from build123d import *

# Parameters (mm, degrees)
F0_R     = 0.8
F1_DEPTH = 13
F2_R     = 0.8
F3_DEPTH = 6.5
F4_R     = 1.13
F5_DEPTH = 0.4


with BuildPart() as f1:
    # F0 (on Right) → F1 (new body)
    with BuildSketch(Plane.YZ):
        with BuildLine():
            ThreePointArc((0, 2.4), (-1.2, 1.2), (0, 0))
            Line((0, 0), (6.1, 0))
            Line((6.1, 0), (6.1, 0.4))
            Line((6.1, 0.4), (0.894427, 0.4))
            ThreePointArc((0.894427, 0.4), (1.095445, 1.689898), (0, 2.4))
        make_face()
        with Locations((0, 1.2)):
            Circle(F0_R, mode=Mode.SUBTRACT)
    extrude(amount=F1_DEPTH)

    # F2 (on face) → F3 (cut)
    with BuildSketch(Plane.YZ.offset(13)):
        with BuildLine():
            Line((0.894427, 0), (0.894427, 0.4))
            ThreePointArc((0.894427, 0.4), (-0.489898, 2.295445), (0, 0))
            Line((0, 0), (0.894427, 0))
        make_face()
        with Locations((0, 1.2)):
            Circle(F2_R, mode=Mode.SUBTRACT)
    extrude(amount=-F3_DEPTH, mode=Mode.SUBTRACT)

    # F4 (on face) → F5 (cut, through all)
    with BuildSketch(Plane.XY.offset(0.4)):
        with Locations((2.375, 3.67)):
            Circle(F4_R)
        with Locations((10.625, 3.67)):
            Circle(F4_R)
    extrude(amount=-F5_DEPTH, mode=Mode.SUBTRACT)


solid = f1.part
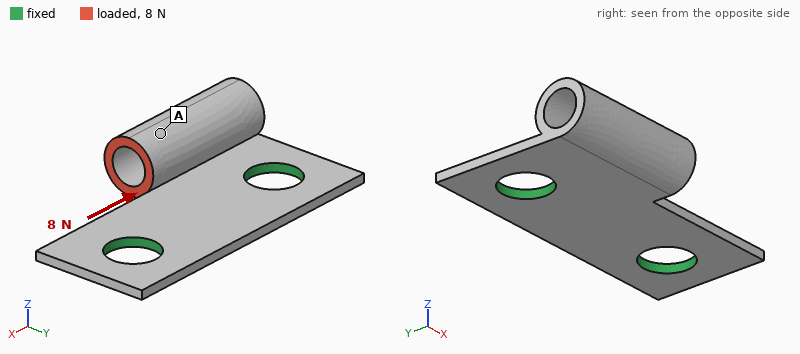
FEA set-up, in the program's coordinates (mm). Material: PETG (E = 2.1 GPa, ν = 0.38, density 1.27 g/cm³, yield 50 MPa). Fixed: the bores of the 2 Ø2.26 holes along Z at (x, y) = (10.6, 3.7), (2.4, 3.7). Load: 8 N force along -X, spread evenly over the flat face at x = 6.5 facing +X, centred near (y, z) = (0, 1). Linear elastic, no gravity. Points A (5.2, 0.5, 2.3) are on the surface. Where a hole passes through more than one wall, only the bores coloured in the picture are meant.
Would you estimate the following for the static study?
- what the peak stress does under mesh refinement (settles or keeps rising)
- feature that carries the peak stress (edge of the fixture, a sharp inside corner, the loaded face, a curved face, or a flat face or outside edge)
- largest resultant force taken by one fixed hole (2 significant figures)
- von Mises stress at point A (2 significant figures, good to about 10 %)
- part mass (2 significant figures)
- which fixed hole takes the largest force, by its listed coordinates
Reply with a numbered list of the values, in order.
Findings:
1. keeps rising
2. a sharp inside corner
3. 5.7 N
4. 3.3 MPa
5. 0.052 g
6. (2.4, 3.7)
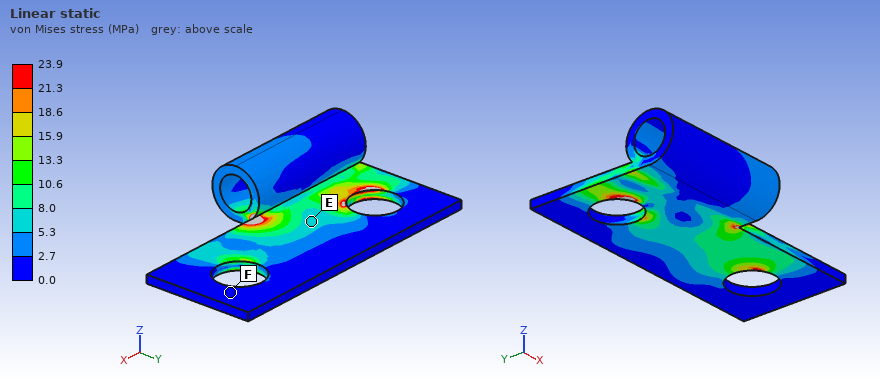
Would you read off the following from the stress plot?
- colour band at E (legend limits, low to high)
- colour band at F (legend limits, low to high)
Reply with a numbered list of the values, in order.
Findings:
1. 5.3 to 8.0 MPa
2. 0.0 to 2.7 MPa
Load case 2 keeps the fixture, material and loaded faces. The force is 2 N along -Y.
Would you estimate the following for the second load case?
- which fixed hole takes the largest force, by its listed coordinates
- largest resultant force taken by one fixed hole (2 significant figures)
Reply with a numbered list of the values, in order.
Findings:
1. (2.4, 3.7)
2. 1.2 N
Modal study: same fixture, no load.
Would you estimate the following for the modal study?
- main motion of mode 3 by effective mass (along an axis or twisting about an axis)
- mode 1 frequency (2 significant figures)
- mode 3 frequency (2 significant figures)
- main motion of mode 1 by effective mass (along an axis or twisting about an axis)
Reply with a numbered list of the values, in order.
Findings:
1. along Z
2. 2900 Hz
3. 12 kHz
4. along Z
